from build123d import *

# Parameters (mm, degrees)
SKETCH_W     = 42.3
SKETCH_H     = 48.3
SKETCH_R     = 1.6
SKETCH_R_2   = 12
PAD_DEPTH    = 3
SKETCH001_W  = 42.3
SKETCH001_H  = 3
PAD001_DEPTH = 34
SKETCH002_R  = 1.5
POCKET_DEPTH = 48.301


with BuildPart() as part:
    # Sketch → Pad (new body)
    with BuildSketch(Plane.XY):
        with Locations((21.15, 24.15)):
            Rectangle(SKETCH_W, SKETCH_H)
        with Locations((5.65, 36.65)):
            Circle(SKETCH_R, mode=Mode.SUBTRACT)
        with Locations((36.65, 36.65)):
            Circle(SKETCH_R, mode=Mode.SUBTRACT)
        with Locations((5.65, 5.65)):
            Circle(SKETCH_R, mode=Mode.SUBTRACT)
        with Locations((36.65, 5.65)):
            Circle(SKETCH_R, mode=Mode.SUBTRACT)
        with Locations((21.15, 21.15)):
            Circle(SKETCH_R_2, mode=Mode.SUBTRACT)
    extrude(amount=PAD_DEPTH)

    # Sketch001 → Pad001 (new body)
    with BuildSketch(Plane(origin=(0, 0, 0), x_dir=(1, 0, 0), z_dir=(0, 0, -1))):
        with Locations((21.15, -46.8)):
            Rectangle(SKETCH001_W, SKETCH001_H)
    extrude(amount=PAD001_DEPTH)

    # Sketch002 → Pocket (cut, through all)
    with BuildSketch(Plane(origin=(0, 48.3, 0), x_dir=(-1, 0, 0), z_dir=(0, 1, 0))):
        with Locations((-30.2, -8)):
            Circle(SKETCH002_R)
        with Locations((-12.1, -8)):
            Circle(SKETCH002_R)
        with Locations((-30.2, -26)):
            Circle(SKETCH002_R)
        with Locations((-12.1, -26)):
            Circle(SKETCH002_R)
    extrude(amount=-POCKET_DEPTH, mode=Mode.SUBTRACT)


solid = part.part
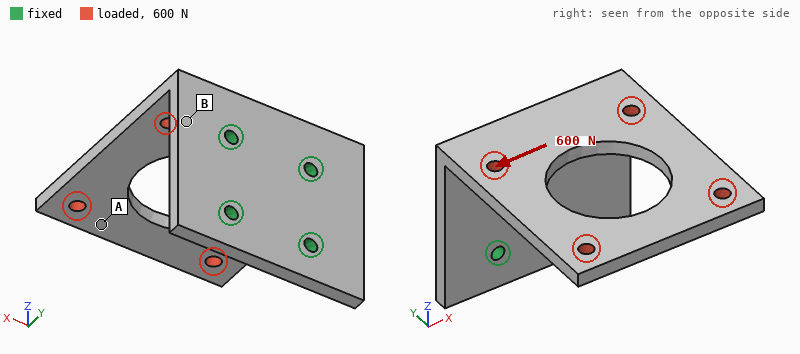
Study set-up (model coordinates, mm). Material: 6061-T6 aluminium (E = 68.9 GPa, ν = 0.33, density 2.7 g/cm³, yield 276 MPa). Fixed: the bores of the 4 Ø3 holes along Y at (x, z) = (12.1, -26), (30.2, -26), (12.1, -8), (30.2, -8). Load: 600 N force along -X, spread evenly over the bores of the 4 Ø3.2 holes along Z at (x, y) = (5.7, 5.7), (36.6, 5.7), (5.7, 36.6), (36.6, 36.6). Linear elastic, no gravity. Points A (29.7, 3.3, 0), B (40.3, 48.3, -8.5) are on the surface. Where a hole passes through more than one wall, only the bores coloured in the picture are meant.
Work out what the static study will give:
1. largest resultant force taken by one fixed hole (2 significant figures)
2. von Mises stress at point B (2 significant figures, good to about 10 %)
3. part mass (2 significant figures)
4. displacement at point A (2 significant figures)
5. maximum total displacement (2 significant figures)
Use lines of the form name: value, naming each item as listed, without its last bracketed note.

largest resultant force taken by one fixed hole: 820 N
von Mises stress at point B: 60 MPa
part mass: 24 g
displacement at point A: 0.22 mm
maximum total displacement: 0.27 mm
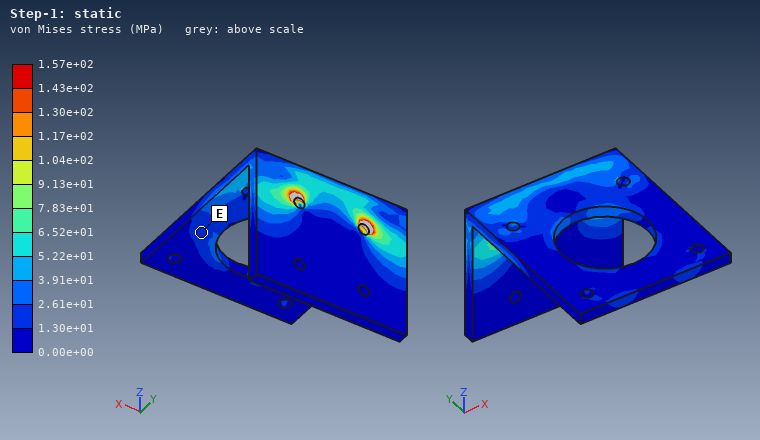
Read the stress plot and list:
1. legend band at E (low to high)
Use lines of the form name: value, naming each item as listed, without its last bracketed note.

legend band at E: 1.30e+01 to 2.61e+01 MPa
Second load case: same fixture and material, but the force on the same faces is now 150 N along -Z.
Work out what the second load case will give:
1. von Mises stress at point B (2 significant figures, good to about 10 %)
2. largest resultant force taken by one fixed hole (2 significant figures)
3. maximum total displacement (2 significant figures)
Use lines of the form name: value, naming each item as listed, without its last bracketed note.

von Mises stress at point B: 31 MPa
largest resultant force taken by one fixed hole: 73 N
maximum total displacement: 0.71 mm
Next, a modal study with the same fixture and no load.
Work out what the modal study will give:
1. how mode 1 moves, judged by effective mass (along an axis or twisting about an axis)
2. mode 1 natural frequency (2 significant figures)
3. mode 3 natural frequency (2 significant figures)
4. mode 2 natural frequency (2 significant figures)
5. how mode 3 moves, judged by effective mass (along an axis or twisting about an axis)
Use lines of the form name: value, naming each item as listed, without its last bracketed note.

how mode 1 moves, judged by effective mass: along Z
mode 1 natural frequency: 870 Hz
mode 3 natural frequency: 3000 Hz
mode 2 natural frequency: 2200 Hz
how mode 3 moves, judged by effective mass: along X
